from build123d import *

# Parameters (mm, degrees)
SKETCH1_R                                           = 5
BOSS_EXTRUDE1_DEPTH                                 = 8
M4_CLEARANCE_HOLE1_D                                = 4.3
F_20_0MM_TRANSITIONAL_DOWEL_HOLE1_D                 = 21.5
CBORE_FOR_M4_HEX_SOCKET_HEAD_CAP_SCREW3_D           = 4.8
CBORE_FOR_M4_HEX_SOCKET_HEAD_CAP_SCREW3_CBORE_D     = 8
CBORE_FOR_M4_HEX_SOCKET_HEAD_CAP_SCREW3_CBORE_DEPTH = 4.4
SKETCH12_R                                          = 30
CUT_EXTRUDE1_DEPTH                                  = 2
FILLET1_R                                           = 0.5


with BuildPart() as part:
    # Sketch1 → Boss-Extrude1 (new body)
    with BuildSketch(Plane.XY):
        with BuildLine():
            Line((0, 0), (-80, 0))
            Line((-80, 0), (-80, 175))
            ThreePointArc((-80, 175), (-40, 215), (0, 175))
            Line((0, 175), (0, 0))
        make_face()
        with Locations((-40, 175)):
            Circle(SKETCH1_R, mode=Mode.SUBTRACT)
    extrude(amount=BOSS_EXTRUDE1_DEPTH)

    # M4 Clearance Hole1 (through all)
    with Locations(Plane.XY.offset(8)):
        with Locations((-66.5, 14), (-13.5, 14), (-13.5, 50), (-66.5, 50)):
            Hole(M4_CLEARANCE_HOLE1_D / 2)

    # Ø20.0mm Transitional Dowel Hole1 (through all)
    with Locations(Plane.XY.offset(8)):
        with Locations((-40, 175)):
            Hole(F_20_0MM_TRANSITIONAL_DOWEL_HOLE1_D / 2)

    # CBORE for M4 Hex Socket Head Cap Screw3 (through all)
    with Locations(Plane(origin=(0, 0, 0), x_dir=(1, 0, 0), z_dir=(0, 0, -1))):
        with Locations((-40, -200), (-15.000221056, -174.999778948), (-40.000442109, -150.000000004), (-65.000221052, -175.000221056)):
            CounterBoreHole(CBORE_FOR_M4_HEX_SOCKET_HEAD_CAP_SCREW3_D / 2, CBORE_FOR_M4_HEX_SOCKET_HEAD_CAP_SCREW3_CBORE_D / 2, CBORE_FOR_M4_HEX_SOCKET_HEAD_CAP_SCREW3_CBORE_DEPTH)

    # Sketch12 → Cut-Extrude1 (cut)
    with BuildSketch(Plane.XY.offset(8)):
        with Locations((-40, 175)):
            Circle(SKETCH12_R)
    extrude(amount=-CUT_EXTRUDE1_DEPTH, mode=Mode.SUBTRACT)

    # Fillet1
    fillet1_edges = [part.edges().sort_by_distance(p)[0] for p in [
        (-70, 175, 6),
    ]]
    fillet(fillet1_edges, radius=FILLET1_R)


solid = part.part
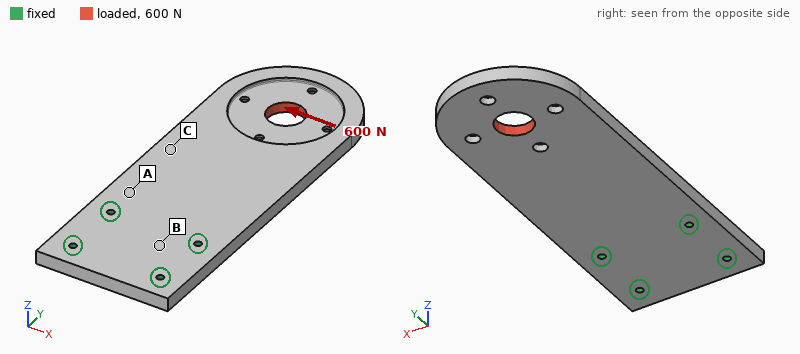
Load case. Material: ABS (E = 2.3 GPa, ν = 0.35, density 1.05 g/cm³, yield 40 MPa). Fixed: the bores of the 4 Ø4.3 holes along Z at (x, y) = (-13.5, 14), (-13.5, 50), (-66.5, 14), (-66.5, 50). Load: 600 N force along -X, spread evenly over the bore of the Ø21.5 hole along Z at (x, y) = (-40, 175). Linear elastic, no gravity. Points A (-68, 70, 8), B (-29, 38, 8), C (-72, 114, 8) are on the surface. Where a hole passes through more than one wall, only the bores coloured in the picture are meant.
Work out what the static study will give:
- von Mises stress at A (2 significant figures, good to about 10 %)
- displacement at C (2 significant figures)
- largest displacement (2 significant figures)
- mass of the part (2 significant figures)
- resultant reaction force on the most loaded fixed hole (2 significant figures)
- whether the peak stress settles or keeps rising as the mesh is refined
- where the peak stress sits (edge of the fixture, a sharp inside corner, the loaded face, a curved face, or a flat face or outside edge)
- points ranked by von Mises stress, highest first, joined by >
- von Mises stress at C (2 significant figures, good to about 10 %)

5.8 MPa
0.35 mm
1.1 mm
130 g
1.1 kN
keeps rising
edge of the fixture
A > C > B
3.3 MPa
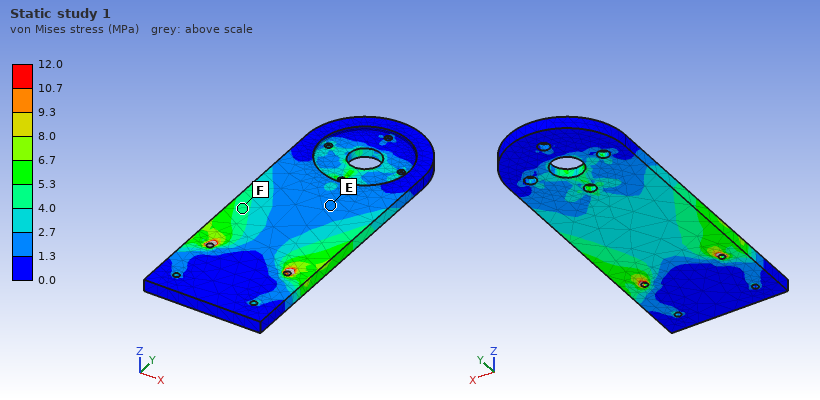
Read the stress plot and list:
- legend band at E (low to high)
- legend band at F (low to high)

1.3 to 2.7 MPa
4.0 to 5.3 MPa
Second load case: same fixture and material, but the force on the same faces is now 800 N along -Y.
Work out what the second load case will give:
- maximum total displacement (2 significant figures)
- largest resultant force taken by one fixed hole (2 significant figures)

1.3 mm
310 N
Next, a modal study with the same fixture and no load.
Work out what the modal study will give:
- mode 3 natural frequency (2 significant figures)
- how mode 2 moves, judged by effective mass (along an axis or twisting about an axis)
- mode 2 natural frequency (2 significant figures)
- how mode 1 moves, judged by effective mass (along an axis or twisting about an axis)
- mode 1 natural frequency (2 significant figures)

430 Hz
twisting about Y
330 Hz
along Z
83 Hz
